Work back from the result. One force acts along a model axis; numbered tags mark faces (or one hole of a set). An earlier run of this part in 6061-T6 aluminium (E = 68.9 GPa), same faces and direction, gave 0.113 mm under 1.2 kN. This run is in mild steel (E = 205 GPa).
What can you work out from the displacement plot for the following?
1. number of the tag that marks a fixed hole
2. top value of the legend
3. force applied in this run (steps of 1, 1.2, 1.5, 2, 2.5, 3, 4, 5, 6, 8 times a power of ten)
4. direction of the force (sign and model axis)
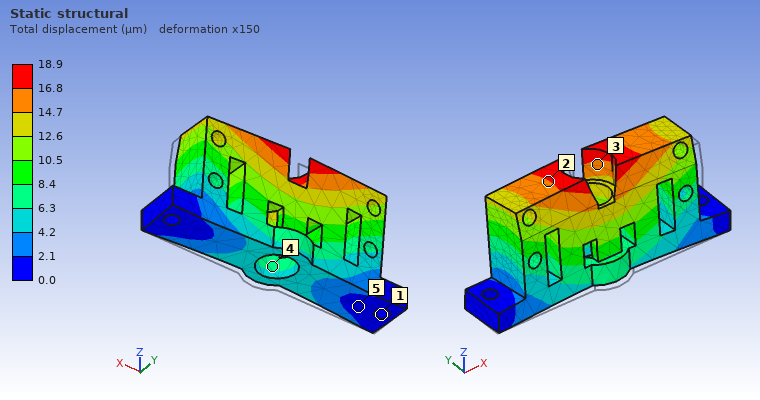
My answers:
1
18.9 µm
600 N
+Y
